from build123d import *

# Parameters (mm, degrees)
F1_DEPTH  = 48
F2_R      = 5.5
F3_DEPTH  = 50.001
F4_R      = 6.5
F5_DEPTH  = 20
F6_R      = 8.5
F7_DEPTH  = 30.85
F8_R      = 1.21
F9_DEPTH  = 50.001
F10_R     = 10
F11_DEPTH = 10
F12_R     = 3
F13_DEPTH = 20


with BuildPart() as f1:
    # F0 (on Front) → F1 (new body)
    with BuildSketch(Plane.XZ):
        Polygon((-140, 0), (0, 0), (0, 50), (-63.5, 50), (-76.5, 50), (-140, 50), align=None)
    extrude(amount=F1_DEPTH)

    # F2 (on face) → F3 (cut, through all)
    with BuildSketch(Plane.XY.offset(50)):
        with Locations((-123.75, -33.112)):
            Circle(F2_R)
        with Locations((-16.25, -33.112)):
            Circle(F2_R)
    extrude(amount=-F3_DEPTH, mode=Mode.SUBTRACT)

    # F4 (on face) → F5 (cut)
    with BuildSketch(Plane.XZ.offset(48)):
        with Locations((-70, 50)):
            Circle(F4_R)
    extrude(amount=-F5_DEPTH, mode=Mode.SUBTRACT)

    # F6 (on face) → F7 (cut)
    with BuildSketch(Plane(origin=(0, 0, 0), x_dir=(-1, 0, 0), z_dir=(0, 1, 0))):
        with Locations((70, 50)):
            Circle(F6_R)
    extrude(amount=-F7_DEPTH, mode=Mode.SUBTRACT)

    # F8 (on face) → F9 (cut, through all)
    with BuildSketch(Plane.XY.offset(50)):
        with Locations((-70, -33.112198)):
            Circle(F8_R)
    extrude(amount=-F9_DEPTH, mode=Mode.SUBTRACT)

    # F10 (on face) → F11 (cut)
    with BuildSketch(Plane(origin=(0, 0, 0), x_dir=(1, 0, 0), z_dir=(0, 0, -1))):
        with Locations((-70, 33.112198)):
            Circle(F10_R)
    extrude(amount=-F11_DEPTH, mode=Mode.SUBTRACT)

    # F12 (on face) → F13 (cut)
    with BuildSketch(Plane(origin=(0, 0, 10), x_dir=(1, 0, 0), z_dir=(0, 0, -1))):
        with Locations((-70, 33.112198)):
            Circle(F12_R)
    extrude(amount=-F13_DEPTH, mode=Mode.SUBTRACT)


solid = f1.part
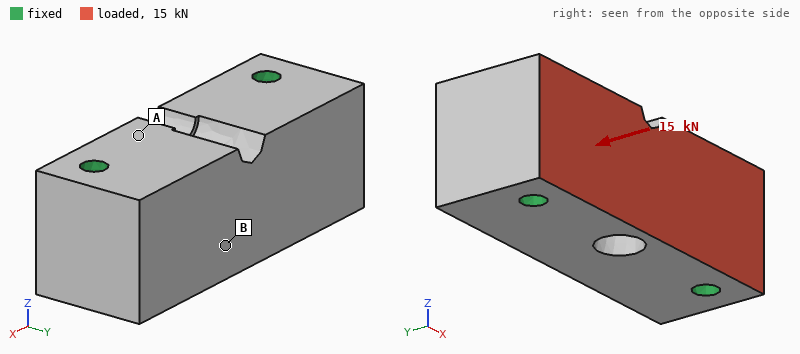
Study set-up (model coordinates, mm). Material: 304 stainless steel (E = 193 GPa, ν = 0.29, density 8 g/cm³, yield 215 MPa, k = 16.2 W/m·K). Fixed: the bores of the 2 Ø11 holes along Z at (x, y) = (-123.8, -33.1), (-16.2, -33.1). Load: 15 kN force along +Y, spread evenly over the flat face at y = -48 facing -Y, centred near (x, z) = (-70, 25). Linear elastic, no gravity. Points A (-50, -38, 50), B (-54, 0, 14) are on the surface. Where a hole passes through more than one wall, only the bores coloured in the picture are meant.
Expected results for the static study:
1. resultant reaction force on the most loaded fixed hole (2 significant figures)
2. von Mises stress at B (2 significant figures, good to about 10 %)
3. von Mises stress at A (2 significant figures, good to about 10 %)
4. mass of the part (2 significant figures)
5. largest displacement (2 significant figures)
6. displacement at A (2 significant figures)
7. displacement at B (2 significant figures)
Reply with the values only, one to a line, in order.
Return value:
7.6 kN
4.8 MPa
2.1 MPa
2.5 kg
2.6 µm
1.7 µm
1.6 µm
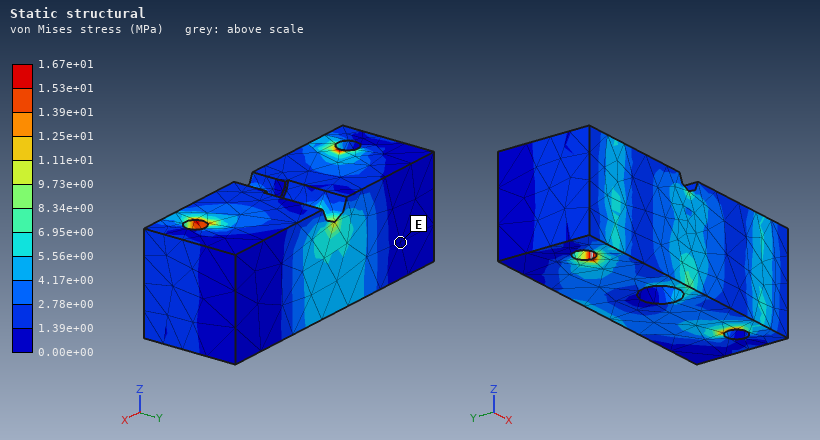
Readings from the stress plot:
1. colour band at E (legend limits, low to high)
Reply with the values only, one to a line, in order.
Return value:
0.00e+00 to 1.39e+00 MPa
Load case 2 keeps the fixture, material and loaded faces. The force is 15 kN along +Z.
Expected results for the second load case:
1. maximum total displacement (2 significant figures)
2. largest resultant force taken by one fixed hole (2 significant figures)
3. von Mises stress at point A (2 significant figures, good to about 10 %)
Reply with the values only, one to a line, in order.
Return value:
4.4 µm
7.5 kN
4.5 MPa
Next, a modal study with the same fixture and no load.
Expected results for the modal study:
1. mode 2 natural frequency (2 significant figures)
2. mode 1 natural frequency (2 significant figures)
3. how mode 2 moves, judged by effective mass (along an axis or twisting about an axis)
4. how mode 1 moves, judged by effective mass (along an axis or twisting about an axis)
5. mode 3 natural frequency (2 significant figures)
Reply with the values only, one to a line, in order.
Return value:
9700 Hz
9200 Hz
along Z
along Y
13 kHz
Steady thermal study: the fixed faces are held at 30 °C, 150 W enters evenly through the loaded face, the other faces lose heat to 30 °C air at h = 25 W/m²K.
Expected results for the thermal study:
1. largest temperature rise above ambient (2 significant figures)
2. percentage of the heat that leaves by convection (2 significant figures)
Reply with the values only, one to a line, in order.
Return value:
64 K
8.5 %
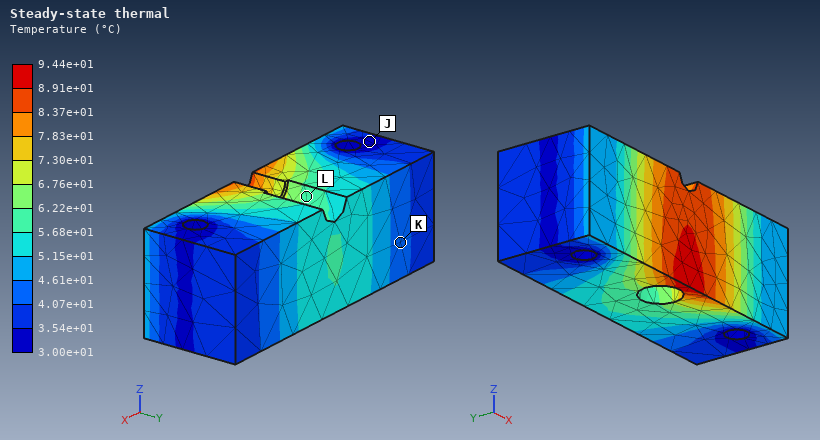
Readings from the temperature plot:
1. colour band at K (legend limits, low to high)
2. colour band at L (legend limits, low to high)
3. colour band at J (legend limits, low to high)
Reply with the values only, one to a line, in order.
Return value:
4.07e+01 to 4.61e+01 °C
5.68e+01 to 6.22e+01 °C
3.00e+01 to 3.54e+01 °C
